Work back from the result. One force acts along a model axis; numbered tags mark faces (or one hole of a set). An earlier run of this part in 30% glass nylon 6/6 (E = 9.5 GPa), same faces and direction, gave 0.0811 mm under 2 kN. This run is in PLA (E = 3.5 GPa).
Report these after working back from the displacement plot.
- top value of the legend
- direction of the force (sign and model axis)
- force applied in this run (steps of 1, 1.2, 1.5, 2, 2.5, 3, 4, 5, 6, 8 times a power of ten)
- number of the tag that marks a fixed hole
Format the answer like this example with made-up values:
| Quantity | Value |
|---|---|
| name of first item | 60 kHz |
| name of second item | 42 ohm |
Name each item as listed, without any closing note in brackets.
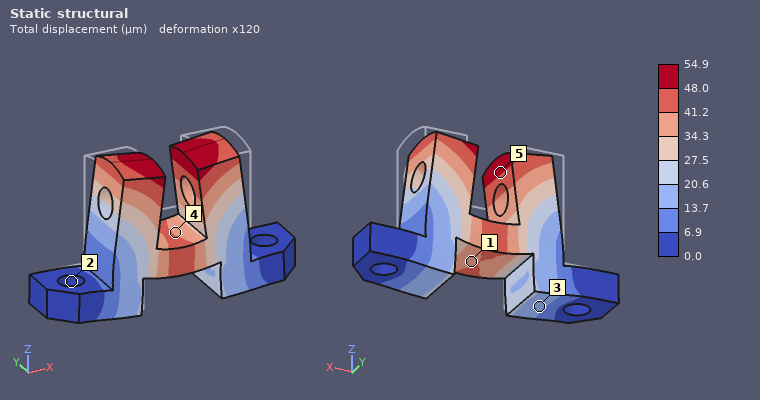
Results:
| Quantity | Value |
|---|---|
| top value of the legend | 54.9 µm |
| direction of the force | -Z |
| force applied in this run | 500 N |
| number of the tag that marks a fixed hole | 2 |
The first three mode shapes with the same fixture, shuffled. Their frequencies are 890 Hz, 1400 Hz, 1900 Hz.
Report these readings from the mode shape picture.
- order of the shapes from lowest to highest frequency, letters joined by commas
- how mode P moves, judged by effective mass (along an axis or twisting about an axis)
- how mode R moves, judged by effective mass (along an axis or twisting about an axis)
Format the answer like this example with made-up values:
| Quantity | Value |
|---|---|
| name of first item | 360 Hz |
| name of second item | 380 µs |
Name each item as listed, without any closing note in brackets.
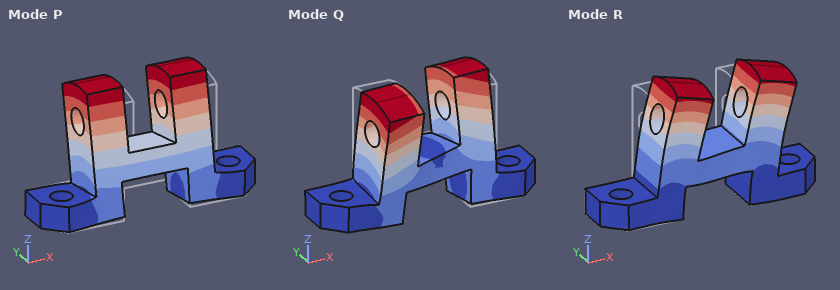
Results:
| Quantity | Value |
|---|---|
| order of the shapes from lowest to highest frequency, letters joined by commas | P, Q, R |
| how mode P moves, judged by effective mass | along Y |
| how mode R moves, judged by effective mass | along X |
